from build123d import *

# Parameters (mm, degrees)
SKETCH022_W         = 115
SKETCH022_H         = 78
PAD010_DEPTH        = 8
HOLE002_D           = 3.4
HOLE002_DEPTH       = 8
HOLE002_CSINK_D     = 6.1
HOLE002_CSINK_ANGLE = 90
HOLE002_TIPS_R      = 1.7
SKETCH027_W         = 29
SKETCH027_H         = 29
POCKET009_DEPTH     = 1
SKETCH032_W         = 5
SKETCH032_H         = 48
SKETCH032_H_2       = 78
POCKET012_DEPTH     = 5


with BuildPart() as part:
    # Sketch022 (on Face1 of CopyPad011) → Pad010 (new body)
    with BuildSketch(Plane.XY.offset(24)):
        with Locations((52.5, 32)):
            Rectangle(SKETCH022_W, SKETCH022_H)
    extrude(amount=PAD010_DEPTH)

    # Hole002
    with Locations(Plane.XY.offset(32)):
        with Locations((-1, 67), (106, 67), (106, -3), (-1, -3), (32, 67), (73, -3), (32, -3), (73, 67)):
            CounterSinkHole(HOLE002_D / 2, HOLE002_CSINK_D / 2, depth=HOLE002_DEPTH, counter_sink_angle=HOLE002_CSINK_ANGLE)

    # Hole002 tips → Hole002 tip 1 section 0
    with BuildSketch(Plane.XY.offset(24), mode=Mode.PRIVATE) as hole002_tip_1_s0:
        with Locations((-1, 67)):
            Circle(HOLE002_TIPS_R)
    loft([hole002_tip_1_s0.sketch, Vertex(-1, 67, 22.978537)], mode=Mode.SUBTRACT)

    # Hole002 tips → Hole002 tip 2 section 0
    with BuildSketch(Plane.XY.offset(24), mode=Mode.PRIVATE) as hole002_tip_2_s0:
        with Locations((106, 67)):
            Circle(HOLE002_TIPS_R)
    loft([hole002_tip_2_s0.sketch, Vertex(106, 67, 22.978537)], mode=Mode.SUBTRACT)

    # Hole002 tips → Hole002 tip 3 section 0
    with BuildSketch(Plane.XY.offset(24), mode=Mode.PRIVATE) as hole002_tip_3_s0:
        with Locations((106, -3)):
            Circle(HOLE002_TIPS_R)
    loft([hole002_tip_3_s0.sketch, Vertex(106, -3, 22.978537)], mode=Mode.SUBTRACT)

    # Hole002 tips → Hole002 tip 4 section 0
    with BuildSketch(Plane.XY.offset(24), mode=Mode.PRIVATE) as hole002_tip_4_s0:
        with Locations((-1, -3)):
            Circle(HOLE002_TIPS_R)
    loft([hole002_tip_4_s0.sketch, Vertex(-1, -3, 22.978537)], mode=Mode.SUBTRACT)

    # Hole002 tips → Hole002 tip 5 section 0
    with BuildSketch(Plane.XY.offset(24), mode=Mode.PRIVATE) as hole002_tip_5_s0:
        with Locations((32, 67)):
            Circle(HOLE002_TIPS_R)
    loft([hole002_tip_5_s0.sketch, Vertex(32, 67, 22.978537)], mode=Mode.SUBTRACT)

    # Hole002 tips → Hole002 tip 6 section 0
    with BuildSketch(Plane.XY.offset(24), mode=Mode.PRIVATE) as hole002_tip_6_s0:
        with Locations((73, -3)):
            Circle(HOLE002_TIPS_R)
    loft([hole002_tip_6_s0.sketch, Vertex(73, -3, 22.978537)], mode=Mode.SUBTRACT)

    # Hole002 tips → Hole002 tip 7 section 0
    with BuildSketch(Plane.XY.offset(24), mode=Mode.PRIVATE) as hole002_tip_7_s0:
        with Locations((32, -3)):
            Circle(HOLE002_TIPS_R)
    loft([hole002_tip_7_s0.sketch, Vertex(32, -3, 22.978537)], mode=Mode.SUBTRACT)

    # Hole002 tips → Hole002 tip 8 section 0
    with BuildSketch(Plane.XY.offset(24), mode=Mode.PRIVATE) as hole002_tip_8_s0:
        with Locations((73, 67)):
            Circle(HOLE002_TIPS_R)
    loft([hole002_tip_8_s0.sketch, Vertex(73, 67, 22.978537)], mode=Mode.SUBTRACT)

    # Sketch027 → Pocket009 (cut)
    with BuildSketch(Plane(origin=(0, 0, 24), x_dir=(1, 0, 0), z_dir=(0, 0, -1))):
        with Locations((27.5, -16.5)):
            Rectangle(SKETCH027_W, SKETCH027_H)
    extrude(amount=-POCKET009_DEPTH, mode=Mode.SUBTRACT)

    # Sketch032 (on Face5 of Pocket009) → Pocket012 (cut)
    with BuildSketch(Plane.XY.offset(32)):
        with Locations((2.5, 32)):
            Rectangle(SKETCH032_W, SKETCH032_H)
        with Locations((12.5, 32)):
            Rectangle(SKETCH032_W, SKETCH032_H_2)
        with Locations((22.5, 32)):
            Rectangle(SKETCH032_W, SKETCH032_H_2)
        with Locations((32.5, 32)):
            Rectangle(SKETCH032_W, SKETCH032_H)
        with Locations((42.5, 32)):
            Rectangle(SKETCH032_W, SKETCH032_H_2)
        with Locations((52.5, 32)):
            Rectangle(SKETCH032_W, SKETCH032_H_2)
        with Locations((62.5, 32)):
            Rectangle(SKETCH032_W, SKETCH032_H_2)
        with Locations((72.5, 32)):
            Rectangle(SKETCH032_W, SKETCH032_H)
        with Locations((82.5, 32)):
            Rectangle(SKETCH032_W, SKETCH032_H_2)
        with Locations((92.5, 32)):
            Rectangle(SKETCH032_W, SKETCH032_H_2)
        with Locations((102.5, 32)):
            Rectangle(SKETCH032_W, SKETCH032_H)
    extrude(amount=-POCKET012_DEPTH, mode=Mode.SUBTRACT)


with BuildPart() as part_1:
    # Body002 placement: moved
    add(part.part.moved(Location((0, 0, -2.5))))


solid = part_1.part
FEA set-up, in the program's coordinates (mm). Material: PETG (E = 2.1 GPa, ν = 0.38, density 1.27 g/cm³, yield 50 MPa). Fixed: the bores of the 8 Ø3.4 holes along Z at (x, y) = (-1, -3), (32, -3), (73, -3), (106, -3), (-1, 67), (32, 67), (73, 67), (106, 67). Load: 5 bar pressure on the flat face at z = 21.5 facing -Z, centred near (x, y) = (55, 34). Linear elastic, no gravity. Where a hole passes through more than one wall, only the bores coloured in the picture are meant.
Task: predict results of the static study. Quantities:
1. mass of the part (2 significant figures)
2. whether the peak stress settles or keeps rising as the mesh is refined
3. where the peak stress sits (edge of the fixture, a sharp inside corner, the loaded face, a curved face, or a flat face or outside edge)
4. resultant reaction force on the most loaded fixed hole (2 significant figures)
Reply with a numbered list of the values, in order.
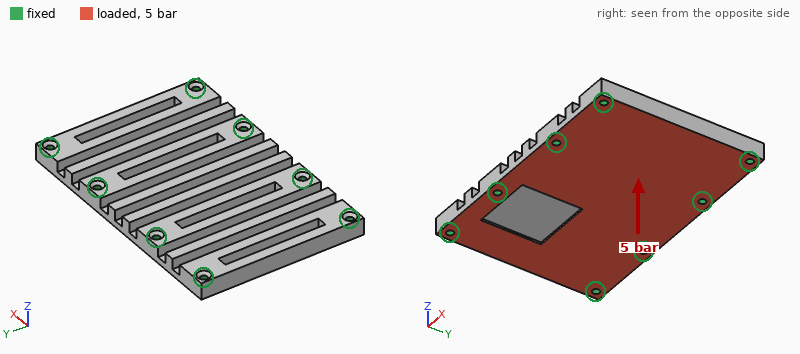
1. 66 g
2. keeps rising
3. edge of the fixture
4. 730 N
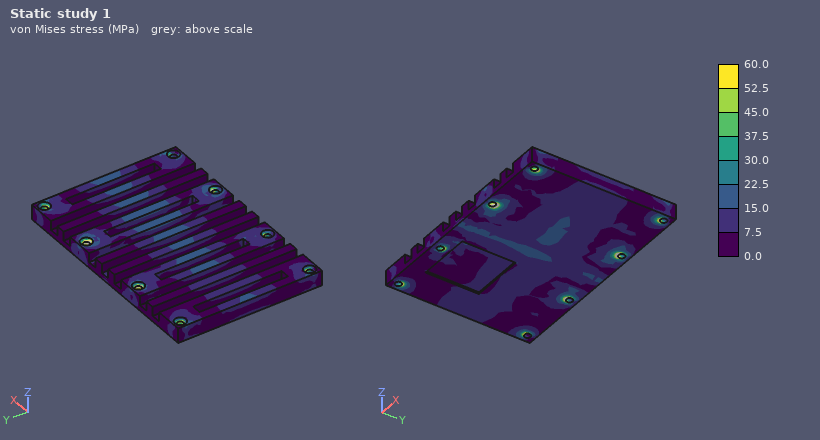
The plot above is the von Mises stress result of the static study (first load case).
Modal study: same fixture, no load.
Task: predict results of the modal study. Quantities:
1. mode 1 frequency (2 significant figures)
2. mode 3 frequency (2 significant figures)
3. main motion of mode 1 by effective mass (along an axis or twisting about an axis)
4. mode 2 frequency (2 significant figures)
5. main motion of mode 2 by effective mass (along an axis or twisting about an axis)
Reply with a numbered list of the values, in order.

1. 1500 Hz
2. 1800 Hz
3. along Z
4. 1700 Hz
5. twisting about Y
